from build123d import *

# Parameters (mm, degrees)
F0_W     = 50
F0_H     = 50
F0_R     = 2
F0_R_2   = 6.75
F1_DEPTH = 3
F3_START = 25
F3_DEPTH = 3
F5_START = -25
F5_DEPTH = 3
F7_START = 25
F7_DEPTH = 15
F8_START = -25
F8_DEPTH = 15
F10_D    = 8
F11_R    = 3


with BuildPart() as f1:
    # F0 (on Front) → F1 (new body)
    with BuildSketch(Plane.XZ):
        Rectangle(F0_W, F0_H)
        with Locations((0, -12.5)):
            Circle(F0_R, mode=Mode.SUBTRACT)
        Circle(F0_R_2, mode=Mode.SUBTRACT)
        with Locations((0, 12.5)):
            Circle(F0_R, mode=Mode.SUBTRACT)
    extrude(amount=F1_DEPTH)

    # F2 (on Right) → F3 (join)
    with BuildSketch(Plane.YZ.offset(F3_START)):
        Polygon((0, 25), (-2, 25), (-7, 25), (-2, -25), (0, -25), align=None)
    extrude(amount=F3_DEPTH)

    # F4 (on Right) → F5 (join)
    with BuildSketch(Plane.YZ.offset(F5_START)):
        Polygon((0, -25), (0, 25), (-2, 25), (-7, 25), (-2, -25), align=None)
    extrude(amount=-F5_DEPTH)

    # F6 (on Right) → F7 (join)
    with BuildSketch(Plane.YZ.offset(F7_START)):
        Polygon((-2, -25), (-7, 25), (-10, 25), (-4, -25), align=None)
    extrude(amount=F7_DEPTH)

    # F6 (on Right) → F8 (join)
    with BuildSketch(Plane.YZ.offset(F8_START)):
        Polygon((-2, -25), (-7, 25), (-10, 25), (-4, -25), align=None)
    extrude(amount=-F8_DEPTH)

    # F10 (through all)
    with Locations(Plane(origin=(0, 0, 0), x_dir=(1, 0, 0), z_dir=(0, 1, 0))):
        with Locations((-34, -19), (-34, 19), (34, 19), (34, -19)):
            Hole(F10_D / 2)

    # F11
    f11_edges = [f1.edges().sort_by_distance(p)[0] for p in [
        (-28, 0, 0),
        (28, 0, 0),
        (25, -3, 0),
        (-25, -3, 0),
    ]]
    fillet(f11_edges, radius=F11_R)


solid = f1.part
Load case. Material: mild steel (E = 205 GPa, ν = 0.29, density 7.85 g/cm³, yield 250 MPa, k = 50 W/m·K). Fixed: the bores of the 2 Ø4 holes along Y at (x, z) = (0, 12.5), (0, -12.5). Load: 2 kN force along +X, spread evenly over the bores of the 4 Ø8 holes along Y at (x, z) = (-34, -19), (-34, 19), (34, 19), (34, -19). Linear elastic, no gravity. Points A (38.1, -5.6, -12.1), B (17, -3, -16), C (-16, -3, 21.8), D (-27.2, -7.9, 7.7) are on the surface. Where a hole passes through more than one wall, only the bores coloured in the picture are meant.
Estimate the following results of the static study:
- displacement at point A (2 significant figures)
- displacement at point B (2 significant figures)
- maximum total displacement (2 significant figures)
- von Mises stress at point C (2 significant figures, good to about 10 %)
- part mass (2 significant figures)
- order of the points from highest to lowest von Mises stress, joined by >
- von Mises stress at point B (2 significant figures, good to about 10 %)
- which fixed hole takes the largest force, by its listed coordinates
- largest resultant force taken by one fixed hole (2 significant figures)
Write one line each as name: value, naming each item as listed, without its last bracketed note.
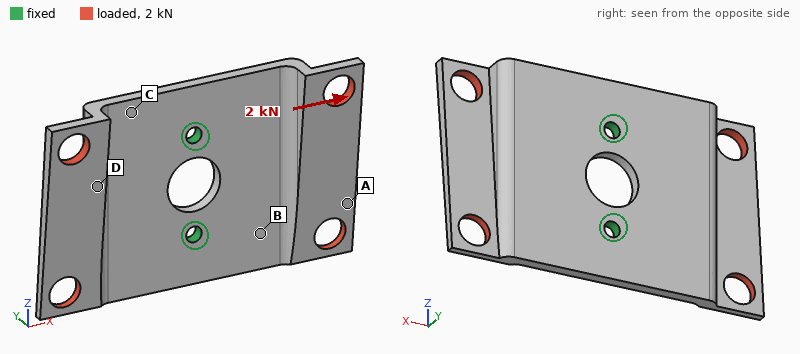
displacement at point A: 0.13 mm
displacement at point B: 0.034 mm
maximum total displacement: 0.19 mm
von Mises stress at point C: 82 MPa
part mass: 91 g
order of the points from highest to lowest von Mises stress, joined by >: C > B > D > A
von Mises stress at point B: 52 MPa
which fixed hole takes the largest force, by its listed coordinates: (0, 12.5)
largest resultant force taken by one fixed hole: 1.2 kN
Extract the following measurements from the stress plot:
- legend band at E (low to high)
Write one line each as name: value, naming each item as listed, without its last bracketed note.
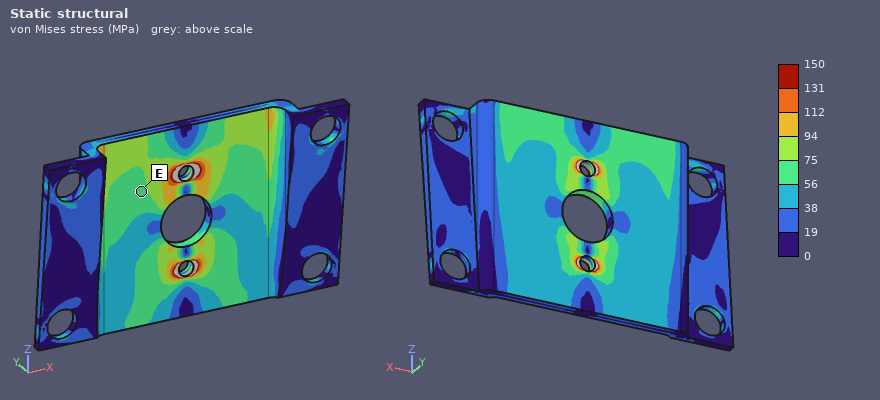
legend band at E: 56 to 75 MPa
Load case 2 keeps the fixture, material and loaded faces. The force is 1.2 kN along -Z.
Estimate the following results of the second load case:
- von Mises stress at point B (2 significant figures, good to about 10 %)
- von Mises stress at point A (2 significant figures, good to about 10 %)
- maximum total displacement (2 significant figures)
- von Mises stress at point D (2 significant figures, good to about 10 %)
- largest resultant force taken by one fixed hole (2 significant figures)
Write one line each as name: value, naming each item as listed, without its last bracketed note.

von Mises stress at point B: 17 MPa
von Mises stress at point A: 5.7 MPa
maximum total displacement: 24 µm
von Mises stress at point D: 13 MPa
largest resultant force taken by one fixed hole: 640 N
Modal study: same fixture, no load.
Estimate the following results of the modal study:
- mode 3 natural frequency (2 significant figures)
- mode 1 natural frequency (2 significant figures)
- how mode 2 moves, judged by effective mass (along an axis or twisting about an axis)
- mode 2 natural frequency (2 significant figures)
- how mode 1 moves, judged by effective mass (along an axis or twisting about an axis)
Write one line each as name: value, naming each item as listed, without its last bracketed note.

mode 3 natural frequency: 3200 Hz
mode 1 natural frequency: 1500 Hz
how mode 2 moves, judged by effective mass: along Y
mode 2 natural frequency: 1600 Hz
how mode 1 moves, judged by effective mass: twisting about Z
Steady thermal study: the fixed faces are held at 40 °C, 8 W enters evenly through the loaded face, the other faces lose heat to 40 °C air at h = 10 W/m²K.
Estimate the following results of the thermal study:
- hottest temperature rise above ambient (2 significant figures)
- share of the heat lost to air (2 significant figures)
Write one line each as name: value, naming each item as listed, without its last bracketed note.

hottest temperature rise above ambient: 30 K
share of the heat lost to air: 14 %
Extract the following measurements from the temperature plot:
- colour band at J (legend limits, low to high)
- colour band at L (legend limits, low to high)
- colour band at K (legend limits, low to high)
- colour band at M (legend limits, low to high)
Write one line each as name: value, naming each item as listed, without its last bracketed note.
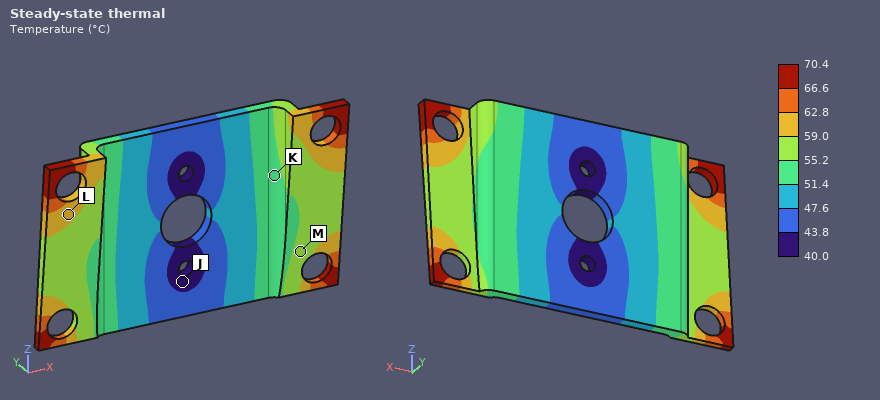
colour band at J: 40.0 to 43.8 °C
colour band at L: 59.0 to 62.8 °C
colour band at K: 51.4 to 55.2 °C
colour band at M: 55.2 to 59.0 °C
